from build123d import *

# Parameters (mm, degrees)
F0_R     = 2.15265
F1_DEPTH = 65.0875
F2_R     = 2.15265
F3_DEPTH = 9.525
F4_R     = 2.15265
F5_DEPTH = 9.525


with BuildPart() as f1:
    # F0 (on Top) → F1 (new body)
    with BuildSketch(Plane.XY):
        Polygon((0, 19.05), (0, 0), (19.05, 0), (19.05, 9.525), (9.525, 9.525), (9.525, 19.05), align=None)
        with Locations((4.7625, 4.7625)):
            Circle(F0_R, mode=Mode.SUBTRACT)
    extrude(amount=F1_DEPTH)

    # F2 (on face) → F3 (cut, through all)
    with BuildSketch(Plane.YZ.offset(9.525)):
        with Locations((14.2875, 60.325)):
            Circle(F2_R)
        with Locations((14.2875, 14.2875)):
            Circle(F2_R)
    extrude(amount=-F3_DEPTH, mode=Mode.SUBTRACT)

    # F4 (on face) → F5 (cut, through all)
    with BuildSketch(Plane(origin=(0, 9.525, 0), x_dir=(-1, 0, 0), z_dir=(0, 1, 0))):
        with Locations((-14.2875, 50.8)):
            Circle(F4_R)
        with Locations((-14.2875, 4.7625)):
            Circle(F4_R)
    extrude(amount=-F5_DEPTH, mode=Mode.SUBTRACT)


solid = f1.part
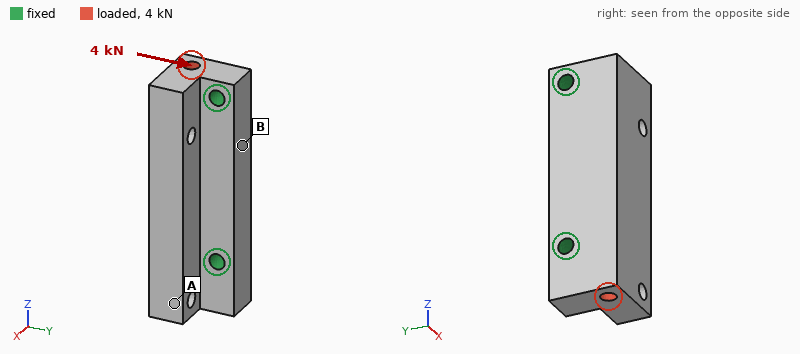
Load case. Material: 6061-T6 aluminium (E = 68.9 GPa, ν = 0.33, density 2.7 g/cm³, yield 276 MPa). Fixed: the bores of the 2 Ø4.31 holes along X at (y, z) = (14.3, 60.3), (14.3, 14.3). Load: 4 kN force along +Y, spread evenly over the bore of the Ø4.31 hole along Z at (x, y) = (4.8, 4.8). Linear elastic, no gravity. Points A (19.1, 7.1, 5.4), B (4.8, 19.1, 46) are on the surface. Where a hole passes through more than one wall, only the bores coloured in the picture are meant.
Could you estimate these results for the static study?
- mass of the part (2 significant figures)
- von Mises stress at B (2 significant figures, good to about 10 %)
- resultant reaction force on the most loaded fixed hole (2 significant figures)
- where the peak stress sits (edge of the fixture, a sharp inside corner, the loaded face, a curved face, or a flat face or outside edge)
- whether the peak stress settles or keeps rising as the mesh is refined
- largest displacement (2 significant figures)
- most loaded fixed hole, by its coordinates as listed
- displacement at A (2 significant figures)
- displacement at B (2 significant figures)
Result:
44 g
9.8 MPa
2.4 kN
edge of the fixture
keeps rising
7.8 µm
(14.3, 14.3)
1.2 µm
6.1 µm
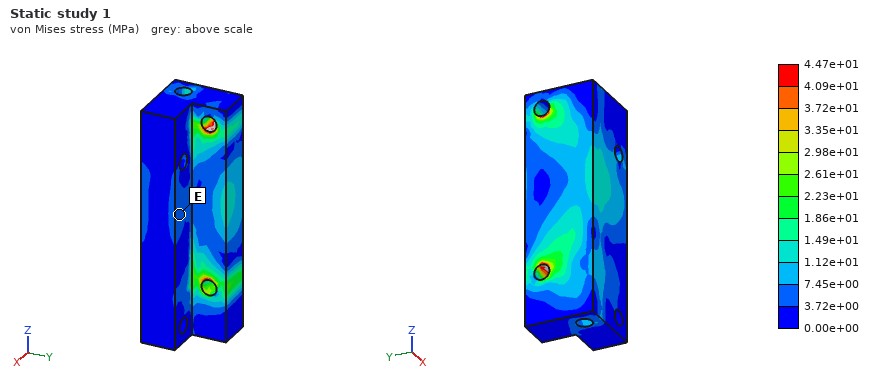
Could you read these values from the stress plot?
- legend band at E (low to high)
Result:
3.72e+00 to 7.45e+00 MPa
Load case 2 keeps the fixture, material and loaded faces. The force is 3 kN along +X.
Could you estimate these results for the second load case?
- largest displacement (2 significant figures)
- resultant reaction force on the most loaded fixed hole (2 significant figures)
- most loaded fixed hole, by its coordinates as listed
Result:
28 µm
1.8 kN
(14.3, 14.3)
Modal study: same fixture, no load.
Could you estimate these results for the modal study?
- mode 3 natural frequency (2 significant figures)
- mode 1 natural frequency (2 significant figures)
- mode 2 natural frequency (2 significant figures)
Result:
19 kHz
11 kHz
16 kHz
